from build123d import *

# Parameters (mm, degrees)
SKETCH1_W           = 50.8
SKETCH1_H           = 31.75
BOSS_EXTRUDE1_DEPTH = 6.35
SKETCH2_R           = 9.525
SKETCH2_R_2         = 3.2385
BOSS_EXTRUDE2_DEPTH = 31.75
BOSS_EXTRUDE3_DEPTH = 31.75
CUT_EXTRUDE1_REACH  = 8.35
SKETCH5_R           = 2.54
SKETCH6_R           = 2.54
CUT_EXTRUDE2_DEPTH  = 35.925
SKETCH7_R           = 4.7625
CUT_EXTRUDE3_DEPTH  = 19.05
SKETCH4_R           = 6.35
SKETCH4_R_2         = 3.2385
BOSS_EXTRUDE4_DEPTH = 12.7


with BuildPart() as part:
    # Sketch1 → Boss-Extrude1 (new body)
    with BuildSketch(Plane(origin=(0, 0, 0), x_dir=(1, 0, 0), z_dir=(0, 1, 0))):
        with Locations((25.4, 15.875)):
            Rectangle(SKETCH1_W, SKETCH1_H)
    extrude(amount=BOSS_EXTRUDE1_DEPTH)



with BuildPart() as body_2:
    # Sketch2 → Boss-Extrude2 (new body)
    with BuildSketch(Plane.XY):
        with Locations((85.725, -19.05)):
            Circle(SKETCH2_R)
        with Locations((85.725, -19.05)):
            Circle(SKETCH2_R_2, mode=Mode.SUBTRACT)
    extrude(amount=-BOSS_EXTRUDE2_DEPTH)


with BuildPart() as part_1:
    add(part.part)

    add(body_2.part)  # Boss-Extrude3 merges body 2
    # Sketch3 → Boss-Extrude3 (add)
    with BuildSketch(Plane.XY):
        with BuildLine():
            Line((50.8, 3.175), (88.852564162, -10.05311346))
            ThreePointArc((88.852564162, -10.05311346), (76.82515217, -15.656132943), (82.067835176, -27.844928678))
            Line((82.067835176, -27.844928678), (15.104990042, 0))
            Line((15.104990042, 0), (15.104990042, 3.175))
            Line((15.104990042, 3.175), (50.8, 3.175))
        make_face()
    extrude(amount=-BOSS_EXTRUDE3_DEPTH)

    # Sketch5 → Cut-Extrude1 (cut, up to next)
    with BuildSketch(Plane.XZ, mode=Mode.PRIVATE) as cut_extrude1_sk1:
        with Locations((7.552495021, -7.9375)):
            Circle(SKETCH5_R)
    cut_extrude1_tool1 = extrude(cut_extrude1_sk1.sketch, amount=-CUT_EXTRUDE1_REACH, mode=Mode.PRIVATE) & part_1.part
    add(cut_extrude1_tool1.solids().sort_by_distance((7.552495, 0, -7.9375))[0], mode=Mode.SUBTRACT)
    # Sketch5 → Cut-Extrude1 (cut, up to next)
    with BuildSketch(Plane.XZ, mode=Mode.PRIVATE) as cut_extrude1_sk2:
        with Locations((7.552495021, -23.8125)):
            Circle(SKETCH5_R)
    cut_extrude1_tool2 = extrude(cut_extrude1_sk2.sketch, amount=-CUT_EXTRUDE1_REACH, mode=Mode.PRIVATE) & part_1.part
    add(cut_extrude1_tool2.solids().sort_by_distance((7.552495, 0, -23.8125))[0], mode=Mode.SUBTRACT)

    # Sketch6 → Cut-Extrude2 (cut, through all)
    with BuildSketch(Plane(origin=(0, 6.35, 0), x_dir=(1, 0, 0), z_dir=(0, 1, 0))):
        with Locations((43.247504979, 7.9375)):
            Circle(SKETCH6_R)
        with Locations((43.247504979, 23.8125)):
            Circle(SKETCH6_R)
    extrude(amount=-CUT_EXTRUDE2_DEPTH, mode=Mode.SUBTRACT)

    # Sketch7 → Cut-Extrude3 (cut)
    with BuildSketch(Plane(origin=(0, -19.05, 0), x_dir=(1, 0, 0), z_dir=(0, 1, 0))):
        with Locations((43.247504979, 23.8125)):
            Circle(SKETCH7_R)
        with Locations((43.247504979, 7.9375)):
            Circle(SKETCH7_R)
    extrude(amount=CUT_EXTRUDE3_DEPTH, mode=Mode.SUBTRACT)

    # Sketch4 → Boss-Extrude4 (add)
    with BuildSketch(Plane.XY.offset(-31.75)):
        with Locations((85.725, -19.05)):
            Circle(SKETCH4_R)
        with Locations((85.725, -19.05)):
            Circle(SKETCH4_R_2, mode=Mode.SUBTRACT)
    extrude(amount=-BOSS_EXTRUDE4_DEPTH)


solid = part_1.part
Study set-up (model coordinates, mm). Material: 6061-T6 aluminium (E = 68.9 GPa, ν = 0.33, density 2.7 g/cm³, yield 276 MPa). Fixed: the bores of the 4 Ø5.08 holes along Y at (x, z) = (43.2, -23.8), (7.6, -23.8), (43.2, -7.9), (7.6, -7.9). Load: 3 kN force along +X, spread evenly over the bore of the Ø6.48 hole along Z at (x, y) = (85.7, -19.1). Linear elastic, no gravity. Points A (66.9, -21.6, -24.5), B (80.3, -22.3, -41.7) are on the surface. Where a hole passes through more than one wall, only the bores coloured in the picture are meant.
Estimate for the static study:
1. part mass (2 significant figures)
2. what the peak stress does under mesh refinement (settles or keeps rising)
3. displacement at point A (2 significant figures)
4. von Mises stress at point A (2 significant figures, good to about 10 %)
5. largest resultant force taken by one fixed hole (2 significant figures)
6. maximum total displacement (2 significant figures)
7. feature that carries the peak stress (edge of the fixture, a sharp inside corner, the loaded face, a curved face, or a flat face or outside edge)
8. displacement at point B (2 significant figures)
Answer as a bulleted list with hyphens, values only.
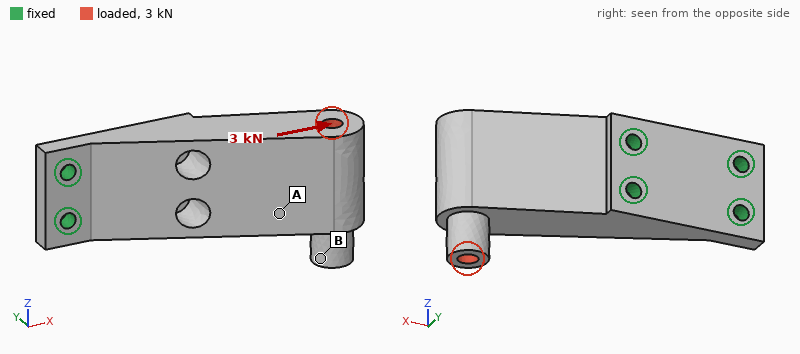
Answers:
- 110 g
- keeps rising
- 0.072 mm
- 19 MPa
- 1.3 kN
- 0.14 mm
- edge of the fixture
- 0.11 mm
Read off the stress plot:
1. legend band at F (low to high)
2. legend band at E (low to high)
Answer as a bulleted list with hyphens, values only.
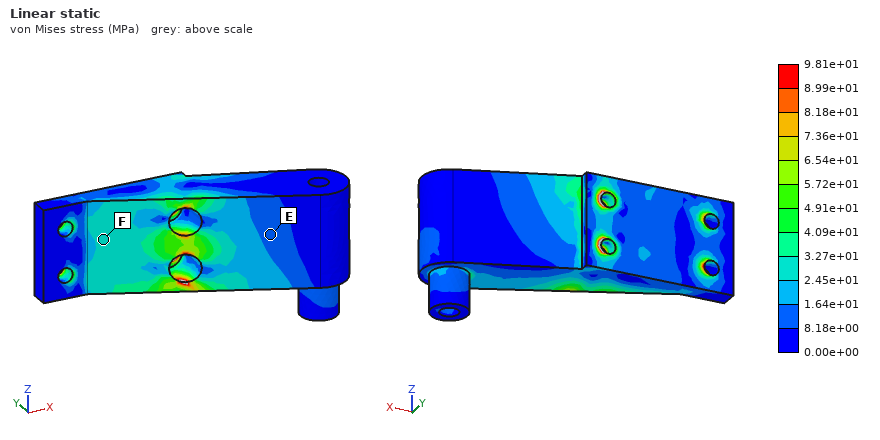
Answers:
- 2.45e+01 to 3.27e+01 MPa
- 8.18e+00 to 1.64e+01 MPa
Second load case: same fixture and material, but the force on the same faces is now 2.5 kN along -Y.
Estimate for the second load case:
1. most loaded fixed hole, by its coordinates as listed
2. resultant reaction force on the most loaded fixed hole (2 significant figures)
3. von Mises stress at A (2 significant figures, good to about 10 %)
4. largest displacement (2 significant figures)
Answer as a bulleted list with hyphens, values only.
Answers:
- (43.2, -23.8)
- 3.5 kN
- 22 MPa
- 0.25 mm
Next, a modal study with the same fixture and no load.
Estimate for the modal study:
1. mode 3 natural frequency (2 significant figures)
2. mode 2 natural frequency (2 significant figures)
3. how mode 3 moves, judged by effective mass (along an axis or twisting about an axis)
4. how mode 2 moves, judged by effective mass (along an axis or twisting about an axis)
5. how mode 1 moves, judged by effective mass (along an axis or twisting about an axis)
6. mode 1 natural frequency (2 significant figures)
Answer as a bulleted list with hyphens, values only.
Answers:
- 8300 Hz
- 4900 Hz
- twisting about X
- along Z
- along Y
- 2900 Hz
